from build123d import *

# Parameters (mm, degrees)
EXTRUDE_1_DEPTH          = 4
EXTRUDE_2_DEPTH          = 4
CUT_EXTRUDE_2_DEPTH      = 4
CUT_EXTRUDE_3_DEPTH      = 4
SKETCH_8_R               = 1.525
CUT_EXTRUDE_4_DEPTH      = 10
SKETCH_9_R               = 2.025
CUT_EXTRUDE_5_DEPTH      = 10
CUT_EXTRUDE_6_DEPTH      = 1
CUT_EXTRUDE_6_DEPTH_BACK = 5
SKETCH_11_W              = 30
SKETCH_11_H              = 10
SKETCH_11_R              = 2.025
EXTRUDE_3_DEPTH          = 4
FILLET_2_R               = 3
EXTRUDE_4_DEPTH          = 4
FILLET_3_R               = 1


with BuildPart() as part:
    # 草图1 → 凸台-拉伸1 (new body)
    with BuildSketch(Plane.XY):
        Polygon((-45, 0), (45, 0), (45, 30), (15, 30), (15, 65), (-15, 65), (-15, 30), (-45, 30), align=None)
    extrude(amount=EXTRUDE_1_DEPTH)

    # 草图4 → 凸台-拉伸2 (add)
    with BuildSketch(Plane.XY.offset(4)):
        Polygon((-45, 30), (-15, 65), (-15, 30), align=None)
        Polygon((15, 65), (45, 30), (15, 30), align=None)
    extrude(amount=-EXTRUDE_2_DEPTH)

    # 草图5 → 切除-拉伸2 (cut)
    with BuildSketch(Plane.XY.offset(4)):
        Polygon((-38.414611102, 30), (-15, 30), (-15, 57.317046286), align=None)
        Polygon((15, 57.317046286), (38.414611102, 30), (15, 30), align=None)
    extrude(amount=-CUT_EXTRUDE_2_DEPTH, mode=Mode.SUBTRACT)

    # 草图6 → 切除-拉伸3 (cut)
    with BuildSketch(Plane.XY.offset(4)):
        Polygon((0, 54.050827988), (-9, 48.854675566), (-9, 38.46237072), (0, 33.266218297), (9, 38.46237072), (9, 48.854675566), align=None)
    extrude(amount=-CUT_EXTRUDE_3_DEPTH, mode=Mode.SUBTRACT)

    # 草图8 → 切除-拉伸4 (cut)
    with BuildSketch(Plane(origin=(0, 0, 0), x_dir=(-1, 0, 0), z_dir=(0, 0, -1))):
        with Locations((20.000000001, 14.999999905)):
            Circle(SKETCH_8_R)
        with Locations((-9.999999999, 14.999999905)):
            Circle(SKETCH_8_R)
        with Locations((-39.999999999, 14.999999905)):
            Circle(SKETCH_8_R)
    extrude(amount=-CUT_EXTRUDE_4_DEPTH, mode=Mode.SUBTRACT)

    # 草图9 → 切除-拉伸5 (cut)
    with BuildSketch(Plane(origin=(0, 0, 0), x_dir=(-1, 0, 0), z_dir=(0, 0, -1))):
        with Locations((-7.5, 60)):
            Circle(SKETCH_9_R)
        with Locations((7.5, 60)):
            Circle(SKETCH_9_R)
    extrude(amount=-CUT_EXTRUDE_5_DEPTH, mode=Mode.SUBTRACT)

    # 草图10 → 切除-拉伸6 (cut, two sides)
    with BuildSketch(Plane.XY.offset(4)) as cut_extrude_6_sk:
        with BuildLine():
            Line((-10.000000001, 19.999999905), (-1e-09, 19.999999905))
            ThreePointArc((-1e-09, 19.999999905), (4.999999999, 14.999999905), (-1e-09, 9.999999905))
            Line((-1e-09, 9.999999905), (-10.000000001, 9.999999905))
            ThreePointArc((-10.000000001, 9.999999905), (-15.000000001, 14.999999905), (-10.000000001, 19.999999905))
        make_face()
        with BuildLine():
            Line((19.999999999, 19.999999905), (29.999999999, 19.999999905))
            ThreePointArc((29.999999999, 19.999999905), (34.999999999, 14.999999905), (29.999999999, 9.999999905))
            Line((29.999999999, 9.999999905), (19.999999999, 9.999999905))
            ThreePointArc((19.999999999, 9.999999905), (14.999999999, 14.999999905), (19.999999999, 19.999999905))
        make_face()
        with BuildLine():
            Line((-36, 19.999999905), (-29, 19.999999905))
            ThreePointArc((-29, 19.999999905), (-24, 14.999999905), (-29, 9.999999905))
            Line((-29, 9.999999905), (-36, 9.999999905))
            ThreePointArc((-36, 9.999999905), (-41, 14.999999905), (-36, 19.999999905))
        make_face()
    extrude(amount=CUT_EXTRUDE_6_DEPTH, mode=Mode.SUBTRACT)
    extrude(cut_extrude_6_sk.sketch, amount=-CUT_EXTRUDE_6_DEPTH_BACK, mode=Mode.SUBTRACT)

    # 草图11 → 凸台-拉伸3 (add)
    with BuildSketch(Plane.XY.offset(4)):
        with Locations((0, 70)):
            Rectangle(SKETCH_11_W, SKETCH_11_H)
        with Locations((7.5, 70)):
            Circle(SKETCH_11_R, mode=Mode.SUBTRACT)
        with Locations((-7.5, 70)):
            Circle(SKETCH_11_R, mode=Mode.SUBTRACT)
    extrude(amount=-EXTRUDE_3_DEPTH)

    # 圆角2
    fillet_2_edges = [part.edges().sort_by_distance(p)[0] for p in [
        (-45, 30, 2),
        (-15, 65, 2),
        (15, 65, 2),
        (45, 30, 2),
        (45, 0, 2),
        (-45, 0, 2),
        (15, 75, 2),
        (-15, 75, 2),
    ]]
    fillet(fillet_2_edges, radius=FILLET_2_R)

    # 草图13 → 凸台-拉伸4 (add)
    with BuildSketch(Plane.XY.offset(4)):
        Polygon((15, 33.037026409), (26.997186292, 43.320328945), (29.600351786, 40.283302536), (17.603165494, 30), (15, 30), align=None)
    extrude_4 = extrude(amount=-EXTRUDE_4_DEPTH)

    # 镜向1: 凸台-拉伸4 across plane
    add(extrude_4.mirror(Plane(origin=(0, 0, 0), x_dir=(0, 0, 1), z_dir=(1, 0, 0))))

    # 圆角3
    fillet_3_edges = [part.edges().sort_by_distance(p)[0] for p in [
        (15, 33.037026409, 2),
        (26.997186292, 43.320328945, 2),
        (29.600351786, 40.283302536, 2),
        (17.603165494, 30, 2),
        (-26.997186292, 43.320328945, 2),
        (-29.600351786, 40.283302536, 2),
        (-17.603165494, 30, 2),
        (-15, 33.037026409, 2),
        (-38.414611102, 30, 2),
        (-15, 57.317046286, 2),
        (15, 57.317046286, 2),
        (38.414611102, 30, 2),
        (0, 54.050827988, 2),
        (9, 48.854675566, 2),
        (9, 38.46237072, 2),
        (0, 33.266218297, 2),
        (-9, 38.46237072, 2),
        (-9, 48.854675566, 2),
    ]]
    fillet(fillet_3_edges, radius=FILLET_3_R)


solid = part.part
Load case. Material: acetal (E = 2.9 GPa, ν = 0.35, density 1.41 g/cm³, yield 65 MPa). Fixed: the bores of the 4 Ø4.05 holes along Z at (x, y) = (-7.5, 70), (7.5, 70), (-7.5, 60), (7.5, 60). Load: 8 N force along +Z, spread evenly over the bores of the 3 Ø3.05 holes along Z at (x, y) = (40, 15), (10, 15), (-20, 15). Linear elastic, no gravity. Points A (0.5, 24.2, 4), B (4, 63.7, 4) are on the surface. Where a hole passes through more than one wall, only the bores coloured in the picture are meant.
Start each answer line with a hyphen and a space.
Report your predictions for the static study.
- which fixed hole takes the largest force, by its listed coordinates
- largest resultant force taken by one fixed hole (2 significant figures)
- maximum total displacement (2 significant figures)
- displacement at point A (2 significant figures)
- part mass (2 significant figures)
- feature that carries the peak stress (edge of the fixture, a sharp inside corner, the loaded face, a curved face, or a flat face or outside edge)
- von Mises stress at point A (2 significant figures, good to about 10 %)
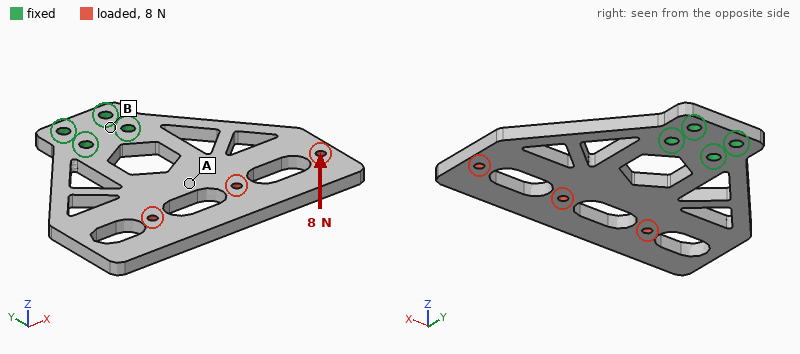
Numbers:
- (7.5, 60)
- 13 N
- 1.1 mm
- 0.44 mm
- 21 g
- a curved face
- 1.0 MPa
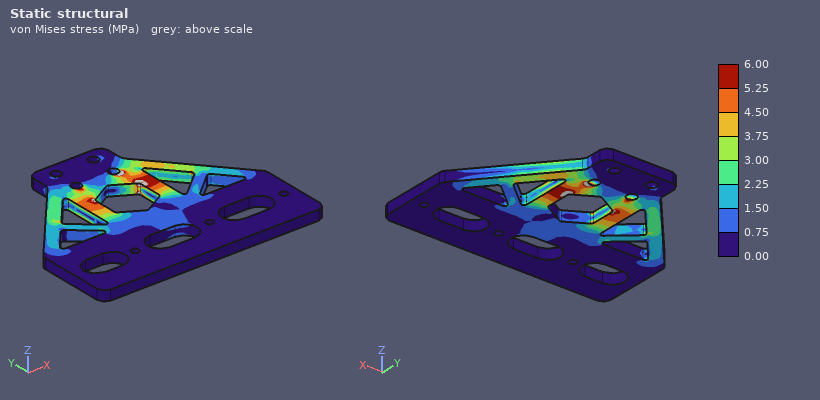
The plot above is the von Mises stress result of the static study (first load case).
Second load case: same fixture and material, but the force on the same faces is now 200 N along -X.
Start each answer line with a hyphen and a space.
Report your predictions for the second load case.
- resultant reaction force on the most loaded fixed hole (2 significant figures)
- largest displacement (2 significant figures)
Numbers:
- 310 N
- 0.91 mm
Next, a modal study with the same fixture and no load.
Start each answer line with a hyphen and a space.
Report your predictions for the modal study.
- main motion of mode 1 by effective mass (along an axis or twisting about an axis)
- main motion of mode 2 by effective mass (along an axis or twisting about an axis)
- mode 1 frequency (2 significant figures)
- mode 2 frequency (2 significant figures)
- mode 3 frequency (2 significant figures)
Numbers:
- along Z
- twisting about Y
- 150 Hz
- 250 Hz
- 690 Hz
